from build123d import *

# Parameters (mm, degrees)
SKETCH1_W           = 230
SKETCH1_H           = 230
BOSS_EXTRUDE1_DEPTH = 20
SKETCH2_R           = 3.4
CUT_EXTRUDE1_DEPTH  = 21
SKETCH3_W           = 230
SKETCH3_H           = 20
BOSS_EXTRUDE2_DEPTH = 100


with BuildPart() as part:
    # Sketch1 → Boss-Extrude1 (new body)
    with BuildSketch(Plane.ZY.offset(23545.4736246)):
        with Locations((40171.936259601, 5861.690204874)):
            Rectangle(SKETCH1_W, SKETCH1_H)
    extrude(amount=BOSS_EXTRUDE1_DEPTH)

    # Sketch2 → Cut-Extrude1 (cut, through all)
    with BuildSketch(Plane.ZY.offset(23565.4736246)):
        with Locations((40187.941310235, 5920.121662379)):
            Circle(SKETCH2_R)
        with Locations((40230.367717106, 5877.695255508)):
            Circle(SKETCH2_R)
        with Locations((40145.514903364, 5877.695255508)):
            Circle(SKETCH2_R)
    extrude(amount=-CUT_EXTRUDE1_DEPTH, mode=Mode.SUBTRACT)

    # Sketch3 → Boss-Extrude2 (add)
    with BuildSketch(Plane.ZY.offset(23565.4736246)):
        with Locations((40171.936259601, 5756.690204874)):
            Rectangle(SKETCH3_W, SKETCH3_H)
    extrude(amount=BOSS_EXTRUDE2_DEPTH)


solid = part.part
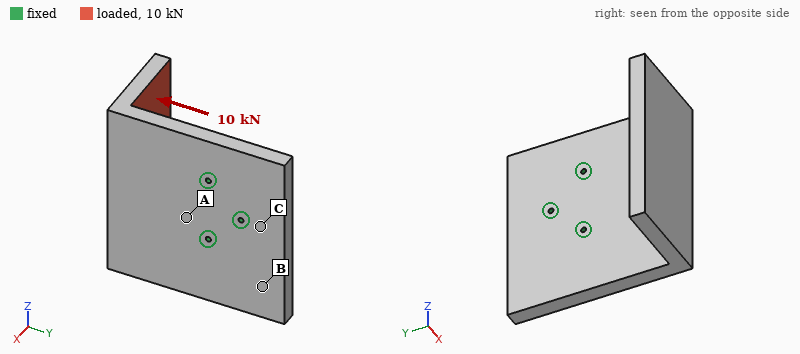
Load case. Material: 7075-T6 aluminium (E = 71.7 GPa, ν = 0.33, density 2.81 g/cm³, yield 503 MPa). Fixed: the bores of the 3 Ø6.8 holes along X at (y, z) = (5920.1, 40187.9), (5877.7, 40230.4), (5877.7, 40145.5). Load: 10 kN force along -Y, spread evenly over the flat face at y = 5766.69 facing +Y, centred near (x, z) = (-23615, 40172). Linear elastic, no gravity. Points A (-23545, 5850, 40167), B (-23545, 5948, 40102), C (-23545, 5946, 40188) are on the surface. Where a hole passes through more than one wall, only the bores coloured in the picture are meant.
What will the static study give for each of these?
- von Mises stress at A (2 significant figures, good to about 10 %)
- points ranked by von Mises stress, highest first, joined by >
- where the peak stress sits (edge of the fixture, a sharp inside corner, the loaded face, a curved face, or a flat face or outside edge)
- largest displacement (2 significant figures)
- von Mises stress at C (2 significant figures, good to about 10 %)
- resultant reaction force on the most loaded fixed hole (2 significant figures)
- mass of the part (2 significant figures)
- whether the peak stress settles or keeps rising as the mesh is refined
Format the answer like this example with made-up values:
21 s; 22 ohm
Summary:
36 MPa; A > C > B; edge of the fixture; 1.1 mm; 15 MPa; 6.2 kN; 4.3 kg; keeps rising
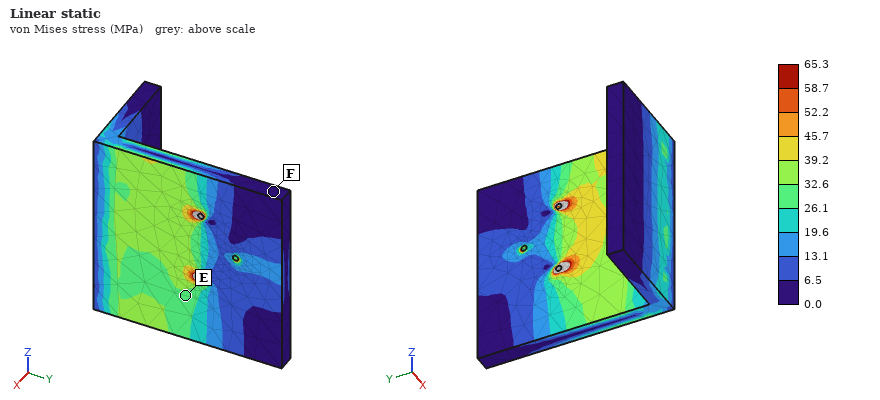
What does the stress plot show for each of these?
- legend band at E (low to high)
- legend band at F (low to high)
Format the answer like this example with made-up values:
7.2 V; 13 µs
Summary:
26.1 to 32.6 MPa; 0.0 to 6.5 MPa
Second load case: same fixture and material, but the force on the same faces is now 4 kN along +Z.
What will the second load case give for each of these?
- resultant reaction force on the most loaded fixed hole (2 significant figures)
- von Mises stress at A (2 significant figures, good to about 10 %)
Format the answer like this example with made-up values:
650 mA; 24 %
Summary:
5.7 kN; 6.3 MPa
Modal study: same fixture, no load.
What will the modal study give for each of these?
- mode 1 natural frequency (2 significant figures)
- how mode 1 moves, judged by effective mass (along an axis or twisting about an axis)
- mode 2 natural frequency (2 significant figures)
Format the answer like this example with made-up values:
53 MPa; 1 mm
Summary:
360 Hz; along X; 590 Hz
